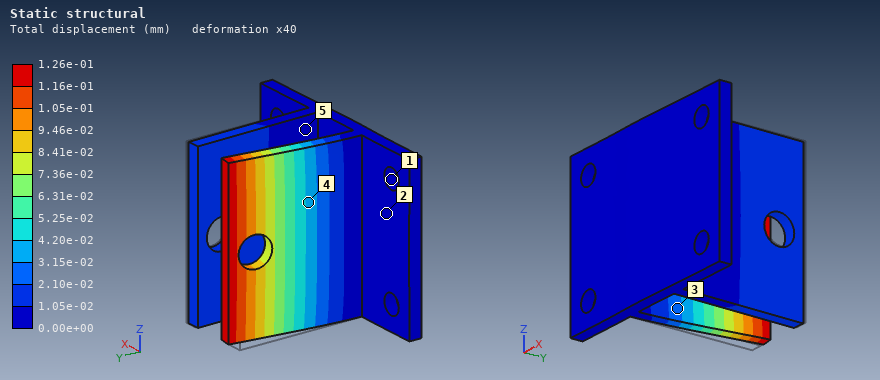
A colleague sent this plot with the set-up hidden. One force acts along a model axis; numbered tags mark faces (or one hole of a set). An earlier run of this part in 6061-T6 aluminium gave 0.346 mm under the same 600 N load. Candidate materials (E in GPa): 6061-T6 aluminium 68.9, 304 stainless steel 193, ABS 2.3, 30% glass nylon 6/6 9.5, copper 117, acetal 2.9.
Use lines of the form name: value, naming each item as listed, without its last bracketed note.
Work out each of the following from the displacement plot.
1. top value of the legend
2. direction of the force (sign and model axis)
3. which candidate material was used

top value of the legend: 1.26e-01 mm
direction of the force: +X
which candidate material was used: 304 stainless steel
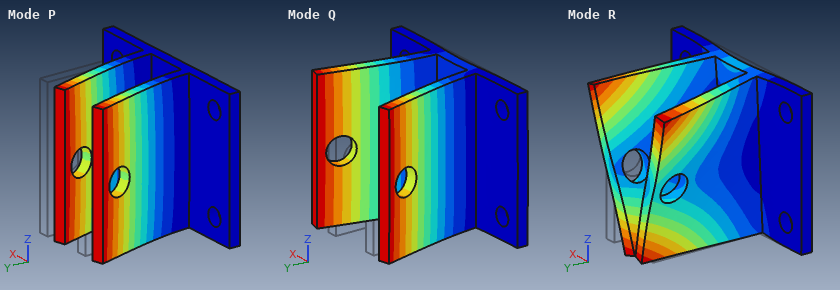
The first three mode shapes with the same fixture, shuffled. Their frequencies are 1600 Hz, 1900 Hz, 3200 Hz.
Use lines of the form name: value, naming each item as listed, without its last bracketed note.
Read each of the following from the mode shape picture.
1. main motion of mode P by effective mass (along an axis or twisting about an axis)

main motion of mode P by effective mass: along X
